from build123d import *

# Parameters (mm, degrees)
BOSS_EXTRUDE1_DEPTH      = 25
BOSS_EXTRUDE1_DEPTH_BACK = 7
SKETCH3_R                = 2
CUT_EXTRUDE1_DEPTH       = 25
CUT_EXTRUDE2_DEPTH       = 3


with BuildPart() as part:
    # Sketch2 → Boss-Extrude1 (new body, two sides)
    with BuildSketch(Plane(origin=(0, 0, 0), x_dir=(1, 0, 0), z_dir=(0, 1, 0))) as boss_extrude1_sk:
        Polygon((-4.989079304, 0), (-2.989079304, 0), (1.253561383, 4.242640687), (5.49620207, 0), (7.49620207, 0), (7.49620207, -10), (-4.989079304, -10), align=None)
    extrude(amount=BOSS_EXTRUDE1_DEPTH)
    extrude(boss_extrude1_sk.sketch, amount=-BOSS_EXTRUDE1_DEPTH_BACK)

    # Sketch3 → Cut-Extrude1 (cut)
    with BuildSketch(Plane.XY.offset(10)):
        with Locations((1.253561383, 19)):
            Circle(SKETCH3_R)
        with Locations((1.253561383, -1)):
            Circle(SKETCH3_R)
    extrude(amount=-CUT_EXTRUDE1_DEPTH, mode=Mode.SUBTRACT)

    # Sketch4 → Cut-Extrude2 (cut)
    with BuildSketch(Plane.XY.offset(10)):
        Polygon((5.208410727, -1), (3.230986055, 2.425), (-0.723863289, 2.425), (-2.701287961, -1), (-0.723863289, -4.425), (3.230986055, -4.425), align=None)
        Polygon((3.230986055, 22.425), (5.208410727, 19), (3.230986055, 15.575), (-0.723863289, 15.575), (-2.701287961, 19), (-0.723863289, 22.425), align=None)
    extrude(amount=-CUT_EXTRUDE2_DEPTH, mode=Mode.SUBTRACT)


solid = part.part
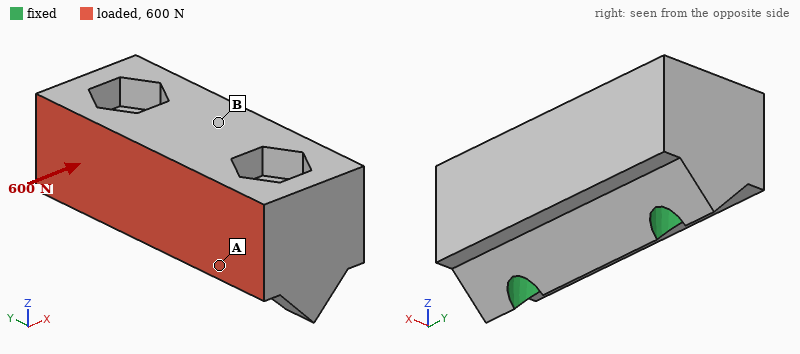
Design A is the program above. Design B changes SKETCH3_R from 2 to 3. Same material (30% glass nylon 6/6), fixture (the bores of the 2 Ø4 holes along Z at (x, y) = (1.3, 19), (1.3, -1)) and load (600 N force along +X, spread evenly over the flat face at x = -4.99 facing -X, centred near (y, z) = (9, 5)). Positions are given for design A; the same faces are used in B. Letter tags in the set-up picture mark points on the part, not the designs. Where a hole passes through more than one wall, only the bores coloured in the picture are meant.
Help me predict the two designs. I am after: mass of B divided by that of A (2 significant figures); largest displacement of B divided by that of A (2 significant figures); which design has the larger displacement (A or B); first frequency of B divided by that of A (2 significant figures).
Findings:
0.93
0.73
A
1.2
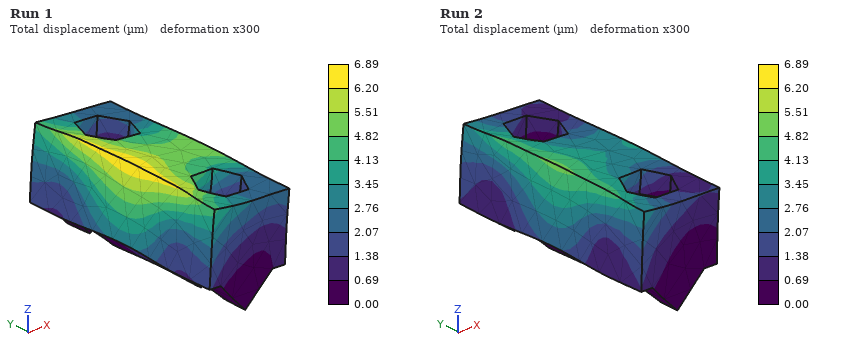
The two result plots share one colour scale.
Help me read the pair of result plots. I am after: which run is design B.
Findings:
Run 2
